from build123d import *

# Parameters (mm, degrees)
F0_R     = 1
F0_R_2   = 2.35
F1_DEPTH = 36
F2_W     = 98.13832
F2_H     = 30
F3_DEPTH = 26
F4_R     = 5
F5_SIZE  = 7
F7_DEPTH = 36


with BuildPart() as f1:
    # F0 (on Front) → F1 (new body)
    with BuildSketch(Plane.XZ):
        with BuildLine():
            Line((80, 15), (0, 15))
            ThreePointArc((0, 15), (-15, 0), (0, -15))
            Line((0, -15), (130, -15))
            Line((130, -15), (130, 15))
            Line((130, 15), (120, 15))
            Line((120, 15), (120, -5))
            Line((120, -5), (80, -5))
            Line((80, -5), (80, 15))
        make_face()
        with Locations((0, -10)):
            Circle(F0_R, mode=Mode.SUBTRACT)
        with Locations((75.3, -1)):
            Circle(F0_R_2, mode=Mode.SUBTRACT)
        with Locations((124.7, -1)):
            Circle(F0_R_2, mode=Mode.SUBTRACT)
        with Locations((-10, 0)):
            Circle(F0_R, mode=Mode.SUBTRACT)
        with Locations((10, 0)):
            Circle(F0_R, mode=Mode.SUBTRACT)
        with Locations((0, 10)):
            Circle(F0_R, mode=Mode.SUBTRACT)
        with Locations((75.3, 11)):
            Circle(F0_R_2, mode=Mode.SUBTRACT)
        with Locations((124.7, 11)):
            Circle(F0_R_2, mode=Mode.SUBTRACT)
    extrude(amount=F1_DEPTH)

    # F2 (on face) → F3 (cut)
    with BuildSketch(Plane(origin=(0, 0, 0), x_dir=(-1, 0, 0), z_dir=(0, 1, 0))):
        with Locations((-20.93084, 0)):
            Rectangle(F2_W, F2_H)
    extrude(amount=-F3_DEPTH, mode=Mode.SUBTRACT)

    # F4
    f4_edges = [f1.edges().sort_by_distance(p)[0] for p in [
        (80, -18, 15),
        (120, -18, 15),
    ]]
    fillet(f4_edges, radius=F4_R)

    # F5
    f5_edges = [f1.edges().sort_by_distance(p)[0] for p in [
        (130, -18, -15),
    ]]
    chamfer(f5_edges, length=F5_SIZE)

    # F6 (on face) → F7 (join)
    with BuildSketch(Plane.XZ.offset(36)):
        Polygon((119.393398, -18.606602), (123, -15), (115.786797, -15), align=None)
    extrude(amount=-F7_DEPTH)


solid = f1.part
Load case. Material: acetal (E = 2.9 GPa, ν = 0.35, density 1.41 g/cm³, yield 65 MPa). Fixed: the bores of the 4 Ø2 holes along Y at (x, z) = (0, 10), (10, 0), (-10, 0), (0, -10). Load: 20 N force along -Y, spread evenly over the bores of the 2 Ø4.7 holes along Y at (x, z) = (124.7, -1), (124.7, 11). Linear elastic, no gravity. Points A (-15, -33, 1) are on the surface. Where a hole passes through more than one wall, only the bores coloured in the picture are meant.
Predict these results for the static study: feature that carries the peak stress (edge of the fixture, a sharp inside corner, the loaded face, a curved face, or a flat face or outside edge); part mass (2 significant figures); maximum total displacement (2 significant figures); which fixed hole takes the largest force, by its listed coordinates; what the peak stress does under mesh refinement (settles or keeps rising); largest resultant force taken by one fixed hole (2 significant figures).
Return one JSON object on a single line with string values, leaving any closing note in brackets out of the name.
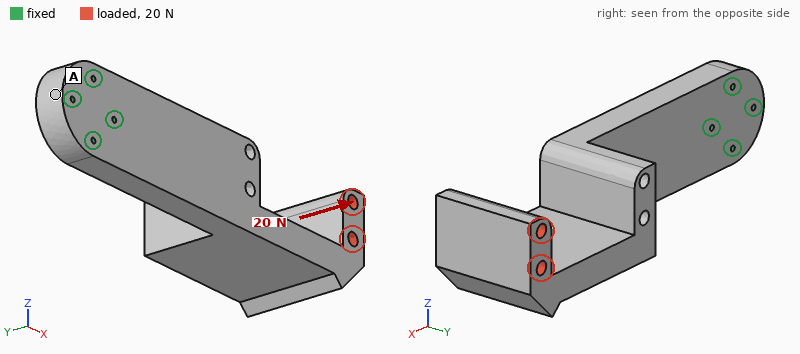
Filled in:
{"feature that carries the peak stress": "edge of the fixture", "part mass": "81 g", "maximum total displacement": "1.6 mm", "which fixed hole takes the largest force, by its listed coordinates": "(10, 0)", "what the peak stress does under mesh refinement": "keeps rising", "largest resultant force taken by one fixed hole": "110 N"}
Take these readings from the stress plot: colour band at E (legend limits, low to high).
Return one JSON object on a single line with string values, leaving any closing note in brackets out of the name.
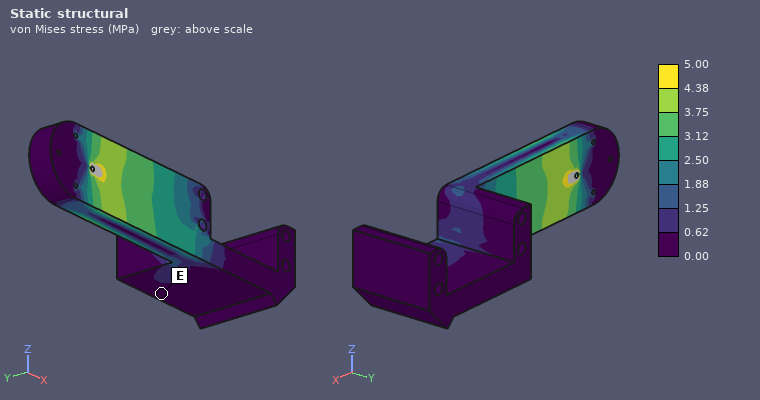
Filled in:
{"colour band at E": "0.00 to 0.62 MPa"}
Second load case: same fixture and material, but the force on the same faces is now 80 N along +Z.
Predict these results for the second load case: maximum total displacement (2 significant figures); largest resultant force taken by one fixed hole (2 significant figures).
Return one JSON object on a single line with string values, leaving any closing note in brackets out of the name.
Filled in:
{"maximum total displacement": "1.7 mm", "largest resultant force taken by one fixed hole": "340 N"}
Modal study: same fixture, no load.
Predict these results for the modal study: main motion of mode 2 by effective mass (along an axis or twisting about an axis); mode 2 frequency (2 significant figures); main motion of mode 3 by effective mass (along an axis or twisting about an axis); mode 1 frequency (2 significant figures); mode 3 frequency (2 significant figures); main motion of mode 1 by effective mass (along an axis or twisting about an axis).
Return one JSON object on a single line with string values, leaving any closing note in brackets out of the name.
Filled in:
{"main motion of mode 2 by effective mass": "along Z", "mode 2 frequency": "240 Hz", "main motion of mode 3 by effective mass": "twisting about X", "mode 1 frequency": "110 Hz", "mode 3 frequency": "570 Hz", "main motion of mode 1 by effective mass": "along Y"}
